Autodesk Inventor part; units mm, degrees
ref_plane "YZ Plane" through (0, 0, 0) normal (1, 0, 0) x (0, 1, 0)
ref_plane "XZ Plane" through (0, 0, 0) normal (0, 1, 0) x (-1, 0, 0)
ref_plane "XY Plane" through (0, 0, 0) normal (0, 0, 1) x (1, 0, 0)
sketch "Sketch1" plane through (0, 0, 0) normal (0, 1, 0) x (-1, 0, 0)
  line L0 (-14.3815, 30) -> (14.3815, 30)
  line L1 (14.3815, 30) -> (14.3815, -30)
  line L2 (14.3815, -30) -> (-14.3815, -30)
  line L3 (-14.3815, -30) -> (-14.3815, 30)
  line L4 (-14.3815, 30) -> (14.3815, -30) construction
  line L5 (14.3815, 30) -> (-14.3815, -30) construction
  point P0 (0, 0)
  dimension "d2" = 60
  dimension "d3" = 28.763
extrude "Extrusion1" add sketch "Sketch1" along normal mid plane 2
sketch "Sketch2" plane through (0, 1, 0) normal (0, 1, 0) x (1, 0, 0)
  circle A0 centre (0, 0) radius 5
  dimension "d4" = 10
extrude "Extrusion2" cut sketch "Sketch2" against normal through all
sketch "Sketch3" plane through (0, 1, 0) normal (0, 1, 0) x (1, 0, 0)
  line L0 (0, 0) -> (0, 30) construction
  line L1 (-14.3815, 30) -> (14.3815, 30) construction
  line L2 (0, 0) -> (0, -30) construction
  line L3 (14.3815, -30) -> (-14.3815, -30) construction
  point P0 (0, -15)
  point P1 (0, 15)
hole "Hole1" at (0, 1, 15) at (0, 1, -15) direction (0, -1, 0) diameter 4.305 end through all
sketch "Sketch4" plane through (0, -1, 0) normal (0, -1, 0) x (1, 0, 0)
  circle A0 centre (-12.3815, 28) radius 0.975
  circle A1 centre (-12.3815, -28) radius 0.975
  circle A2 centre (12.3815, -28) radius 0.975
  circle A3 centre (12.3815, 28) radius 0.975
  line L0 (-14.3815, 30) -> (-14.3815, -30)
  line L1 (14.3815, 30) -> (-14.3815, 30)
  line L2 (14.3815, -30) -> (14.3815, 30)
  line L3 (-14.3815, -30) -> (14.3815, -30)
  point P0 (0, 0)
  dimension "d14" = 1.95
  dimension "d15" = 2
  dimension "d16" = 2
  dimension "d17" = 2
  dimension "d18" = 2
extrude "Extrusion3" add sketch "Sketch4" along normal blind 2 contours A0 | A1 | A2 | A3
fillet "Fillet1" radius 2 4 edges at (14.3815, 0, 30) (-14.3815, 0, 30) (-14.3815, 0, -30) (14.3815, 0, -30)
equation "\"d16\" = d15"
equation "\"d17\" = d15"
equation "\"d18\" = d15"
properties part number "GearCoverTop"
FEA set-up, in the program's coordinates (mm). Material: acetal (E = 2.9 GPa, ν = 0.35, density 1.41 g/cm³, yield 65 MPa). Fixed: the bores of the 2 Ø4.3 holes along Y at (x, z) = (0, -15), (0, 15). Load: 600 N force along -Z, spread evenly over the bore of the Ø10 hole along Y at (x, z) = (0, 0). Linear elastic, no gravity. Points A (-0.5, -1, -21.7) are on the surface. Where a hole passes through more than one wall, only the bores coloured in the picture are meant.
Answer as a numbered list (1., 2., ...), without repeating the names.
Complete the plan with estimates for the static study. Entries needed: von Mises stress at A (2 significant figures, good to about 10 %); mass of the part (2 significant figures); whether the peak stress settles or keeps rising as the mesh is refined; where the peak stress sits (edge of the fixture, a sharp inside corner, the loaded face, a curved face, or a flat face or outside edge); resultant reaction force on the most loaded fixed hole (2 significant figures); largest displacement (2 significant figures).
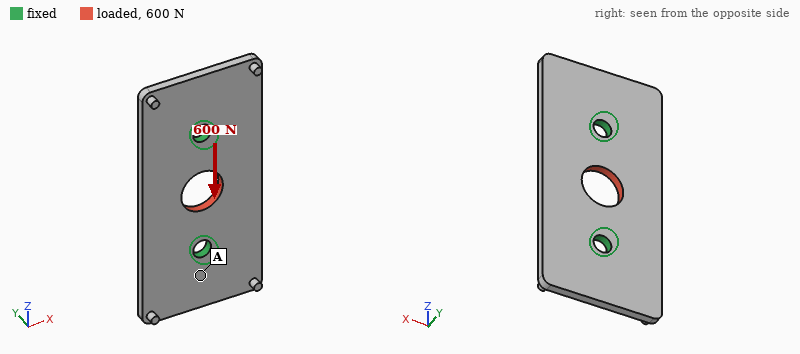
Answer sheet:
1. 2.6 MPa
2. 4.6 g
3. keeps rising
4. edge of the fixture
5. 300 N
6. 52 µm
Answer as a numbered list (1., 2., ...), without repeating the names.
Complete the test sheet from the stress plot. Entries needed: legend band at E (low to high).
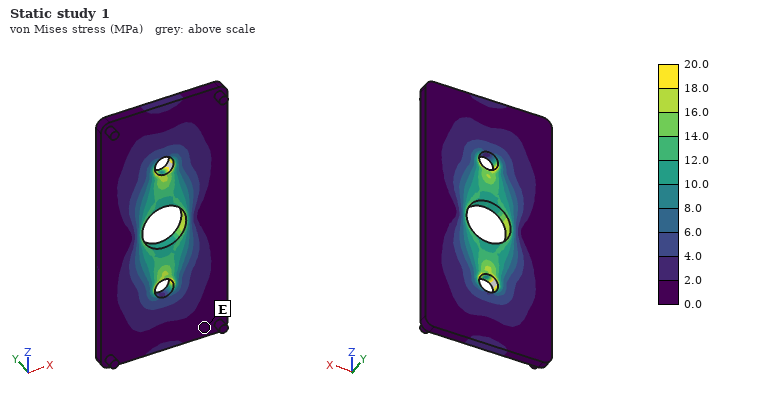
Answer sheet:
1. 0.0 to 2.0 MPa
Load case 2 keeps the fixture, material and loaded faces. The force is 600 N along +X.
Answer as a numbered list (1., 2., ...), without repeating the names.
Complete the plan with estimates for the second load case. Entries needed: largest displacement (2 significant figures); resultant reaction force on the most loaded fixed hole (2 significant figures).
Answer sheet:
1. 0.10 mm
2. 300 N
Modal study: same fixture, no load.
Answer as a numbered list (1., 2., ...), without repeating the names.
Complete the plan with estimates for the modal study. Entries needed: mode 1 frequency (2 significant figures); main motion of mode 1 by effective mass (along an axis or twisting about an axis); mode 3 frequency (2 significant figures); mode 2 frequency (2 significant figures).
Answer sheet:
1. 1800 Hz
2. twisting about Z
3. 1900 Hz
4. 1900 Hz
